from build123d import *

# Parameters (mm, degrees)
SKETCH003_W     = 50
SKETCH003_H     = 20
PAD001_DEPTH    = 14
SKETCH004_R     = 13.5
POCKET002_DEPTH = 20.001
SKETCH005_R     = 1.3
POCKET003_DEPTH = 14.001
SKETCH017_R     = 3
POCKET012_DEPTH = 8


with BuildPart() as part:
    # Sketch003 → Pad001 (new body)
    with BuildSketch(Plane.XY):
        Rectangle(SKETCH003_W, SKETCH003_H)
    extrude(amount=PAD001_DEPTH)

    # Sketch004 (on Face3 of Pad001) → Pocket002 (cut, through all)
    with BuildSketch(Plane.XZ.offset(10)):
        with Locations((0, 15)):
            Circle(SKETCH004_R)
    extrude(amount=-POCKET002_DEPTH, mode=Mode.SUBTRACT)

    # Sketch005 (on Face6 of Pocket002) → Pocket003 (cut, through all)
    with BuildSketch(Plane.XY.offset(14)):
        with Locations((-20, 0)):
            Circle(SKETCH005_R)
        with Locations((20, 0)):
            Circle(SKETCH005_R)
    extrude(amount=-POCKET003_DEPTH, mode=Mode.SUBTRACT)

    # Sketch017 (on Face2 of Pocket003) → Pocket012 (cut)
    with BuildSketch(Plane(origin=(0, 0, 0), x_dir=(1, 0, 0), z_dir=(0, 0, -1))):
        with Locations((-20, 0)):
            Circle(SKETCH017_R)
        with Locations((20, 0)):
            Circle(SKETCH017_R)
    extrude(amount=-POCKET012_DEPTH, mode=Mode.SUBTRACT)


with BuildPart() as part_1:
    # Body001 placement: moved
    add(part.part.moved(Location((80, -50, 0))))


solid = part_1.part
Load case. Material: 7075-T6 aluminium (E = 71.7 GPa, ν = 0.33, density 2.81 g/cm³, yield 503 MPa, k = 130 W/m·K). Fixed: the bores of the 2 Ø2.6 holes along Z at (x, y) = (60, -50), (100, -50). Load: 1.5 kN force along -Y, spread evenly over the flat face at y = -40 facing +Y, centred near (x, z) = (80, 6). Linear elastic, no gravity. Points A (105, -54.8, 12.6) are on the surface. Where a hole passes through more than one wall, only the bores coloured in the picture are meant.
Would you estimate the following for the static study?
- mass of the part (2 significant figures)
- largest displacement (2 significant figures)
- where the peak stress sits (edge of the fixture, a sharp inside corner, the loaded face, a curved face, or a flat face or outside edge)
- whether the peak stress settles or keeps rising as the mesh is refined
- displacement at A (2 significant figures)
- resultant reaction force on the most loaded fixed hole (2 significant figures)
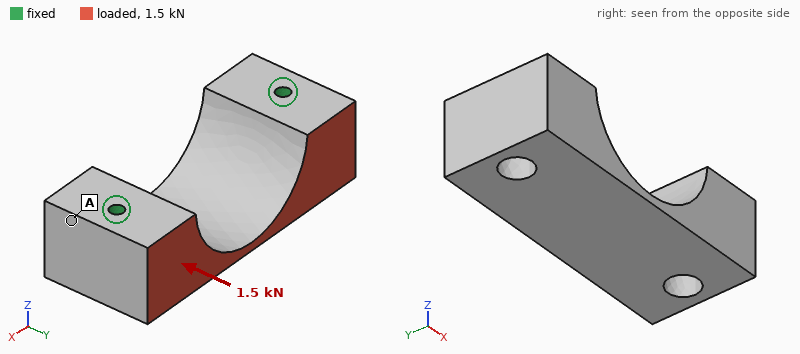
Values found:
23 g
16 µm
edge of the fixture
keeps rising
3.2 µm
750 N
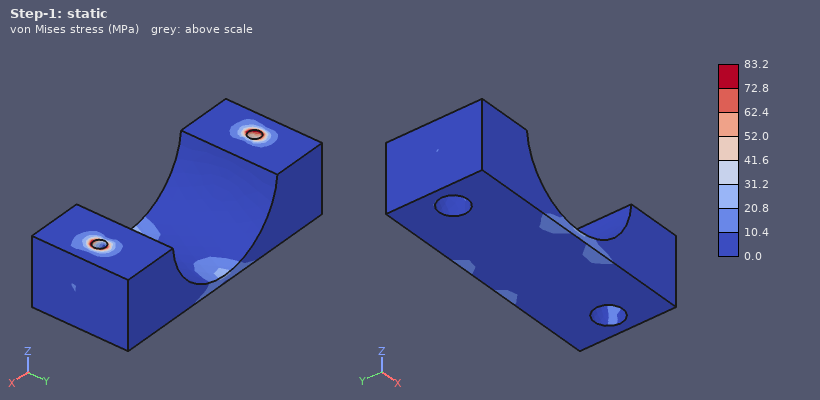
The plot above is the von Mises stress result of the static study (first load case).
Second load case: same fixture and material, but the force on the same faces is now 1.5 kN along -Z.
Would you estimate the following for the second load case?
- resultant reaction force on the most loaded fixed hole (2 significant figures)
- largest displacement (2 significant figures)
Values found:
770 N
28 µm
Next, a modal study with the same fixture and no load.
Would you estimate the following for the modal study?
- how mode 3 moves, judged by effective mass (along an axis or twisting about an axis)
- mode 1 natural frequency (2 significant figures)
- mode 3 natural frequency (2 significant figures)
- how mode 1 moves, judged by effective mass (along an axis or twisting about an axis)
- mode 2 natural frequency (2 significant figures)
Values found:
along X
12 kHz
16 kHz
along Y
15 kHz
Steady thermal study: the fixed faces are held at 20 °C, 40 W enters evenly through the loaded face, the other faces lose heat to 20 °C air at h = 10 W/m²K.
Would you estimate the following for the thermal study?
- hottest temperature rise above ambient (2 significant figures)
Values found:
16 K
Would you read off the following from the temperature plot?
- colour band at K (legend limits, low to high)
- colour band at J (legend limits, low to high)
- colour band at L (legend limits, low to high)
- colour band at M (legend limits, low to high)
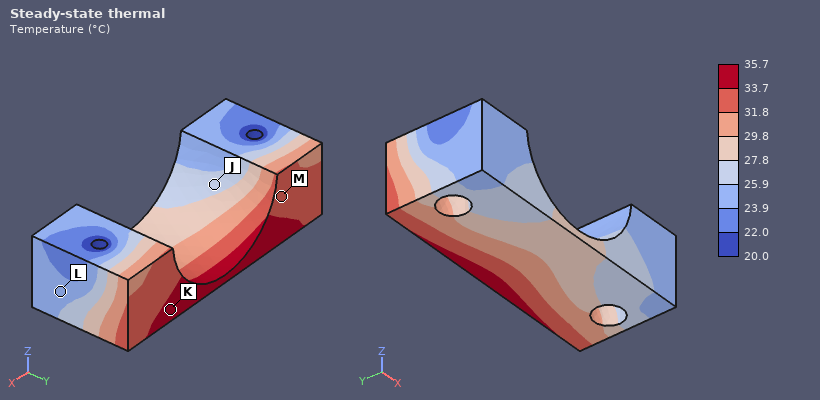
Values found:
33.7 to 35.7 °C
25.9 to 27.8 °C
23.9 to 25.9 °C
31.8 to 33.7 °C
